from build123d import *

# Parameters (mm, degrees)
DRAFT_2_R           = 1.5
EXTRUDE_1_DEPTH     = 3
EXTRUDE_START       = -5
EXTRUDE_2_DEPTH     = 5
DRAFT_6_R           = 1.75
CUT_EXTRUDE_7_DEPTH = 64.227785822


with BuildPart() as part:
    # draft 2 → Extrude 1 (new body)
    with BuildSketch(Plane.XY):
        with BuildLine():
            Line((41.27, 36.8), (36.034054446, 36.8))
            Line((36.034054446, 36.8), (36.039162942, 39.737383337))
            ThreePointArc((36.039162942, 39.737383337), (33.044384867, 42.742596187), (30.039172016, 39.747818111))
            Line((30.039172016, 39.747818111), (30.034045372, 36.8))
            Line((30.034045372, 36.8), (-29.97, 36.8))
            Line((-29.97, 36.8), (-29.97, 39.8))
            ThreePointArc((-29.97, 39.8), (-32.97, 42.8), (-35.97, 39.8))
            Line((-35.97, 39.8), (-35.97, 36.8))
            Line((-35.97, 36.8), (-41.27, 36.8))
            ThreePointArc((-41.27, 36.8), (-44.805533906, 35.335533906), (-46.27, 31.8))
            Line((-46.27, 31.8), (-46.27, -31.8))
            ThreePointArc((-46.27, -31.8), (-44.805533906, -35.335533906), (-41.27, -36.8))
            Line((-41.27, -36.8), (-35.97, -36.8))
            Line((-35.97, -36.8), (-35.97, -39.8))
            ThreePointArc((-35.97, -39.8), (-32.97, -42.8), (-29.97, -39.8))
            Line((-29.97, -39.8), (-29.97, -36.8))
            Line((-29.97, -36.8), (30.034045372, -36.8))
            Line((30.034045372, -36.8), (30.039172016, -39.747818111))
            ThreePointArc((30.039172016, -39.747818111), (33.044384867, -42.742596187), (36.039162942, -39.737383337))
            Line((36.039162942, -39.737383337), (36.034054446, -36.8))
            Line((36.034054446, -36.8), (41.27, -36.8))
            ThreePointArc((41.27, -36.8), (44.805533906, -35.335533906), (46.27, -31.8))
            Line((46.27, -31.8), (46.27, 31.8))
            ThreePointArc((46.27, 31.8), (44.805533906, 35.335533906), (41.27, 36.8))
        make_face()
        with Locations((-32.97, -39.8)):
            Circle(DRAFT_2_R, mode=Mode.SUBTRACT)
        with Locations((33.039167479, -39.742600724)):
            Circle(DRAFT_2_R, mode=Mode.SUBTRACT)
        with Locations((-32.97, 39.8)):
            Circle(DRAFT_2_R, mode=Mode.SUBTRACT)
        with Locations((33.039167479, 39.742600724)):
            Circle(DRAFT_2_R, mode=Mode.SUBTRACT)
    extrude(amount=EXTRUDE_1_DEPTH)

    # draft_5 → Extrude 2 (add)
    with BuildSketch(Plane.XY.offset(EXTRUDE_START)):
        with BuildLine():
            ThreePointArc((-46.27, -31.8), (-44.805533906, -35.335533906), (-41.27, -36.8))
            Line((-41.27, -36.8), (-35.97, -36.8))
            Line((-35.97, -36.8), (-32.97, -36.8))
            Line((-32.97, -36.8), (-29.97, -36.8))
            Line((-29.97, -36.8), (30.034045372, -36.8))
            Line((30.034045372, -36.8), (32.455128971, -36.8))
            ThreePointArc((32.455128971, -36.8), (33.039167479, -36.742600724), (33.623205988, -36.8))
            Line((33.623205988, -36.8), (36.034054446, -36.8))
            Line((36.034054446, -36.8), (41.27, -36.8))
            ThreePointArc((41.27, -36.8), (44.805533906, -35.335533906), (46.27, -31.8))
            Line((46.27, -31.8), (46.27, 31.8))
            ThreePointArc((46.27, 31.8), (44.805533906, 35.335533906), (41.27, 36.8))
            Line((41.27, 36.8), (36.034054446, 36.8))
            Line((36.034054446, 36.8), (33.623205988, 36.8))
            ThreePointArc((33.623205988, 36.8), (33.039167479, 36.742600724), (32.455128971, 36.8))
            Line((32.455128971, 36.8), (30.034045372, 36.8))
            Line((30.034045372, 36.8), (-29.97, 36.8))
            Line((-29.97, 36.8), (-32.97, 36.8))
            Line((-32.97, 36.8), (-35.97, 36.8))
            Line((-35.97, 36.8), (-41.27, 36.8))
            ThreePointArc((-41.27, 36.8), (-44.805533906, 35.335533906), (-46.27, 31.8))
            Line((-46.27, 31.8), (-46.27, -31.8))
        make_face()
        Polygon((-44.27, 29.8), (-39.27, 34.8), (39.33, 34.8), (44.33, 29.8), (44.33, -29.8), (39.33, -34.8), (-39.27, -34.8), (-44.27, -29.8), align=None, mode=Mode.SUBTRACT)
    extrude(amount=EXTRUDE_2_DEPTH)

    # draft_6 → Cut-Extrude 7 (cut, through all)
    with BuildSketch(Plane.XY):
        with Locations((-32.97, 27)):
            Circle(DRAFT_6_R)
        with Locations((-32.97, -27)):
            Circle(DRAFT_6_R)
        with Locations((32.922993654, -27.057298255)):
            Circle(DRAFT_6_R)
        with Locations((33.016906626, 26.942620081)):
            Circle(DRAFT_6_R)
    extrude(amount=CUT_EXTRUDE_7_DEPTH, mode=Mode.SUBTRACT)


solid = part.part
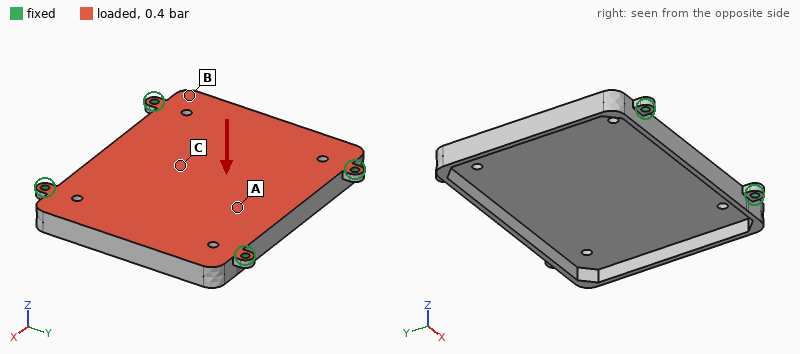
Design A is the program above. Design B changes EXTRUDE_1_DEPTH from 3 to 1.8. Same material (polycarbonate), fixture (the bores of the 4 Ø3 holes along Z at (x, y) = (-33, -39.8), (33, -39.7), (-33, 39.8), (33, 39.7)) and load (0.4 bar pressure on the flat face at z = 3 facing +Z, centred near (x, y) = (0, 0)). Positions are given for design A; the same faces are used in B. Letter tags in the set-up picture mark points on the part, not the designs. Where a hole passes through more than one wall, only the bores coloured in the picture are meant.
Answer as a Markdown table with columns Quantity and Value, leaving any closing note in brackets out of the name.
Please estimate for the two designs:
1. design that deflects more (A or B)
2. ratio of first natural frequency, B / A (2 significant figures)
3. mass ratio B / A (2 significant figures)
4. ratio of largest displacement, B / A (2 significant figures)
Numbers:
| Quantity | Value |
|---|---|
| design that deflects more | B |
| ratio of first natural frequency, B / A | 0.71 |
| mass ratio B / A | 0.66 |
| ratio of largest displacement, B / A | 3.5 |
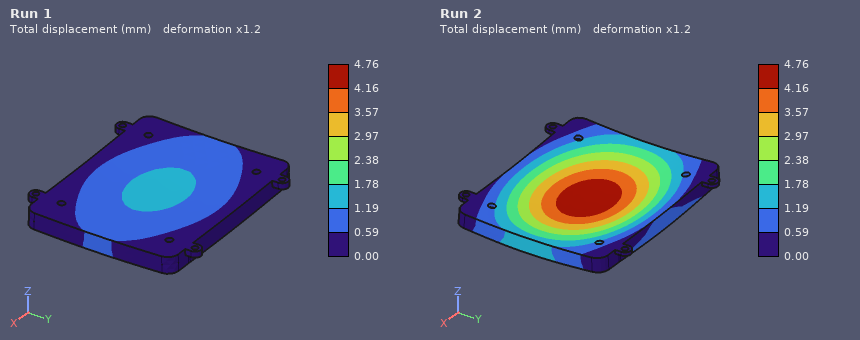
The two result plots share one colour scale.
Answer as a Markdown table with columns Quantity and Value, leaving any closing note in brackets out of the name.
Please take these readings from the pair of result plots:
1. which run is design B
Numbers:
| Quantity | Value |
|---|---|
| which run is design B | Run 2 |
